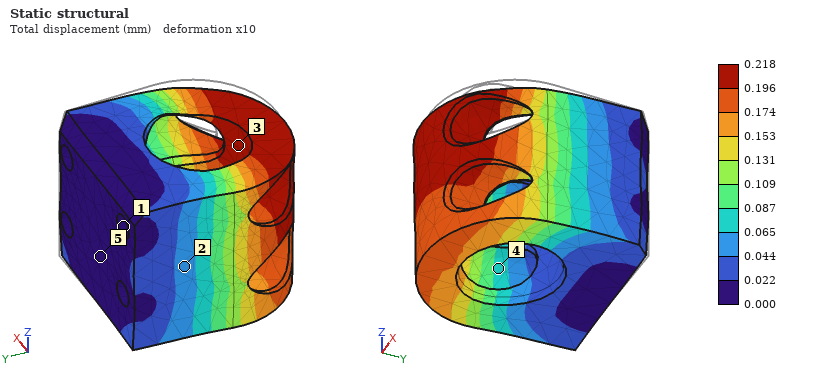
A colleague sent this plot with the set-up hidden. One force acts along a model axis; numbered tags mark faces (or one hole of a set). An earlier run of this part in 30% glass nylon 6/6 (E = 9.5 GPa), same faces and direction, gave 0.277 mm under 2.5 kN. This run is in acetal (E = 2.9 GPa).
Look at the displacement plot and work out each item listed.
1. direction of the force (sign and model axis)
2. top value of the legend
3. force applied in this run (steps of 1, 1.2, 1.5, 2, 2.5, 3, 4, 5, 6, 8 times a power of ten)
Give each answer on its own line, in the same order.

-X
0.218 mm
600 N
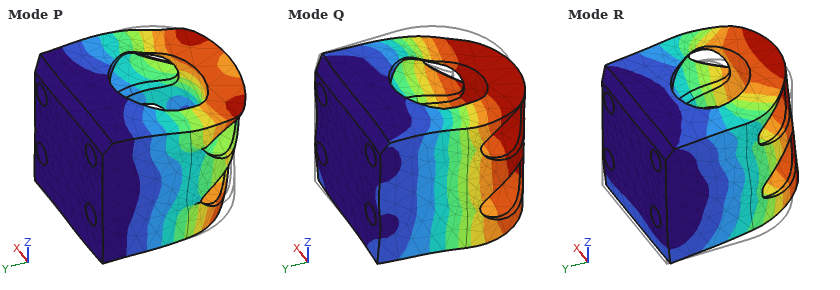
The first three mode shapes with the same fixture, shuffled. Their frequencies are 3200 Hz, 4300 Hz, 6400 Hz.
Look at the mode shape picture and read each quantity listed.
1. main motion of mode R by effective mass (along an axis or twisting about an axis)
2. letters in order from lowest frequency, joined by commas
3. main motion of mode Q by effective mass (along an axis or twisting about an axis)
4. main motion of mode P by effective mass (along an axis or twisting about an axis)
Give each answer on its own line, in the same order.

along Z
R, Q, P
along X
twisting about Y
